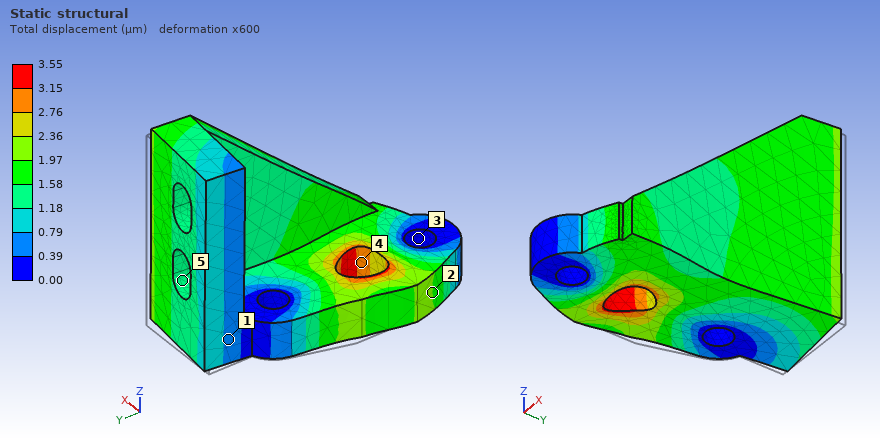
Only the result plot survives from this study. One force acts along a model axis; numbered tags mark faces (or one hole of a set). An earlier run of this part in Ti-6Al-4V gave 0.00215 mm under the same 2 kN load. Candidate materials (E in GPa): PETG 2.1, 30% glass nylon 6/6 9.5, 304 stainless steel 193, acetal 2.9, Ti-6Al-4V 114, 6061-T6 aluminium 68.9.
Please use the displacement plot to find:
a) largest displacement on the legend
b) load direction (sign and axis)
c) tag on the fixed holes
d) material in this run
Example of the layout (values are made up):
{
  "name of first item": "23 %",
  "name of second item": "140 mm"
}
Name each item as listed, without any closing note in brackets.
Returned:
{
  "largest displacement on the legend": "3.55 µm",
  "load direction": "-Y",
  "tag on the fixed holes": "3",
  "material in this run": "6061-T6 aluminium"
}
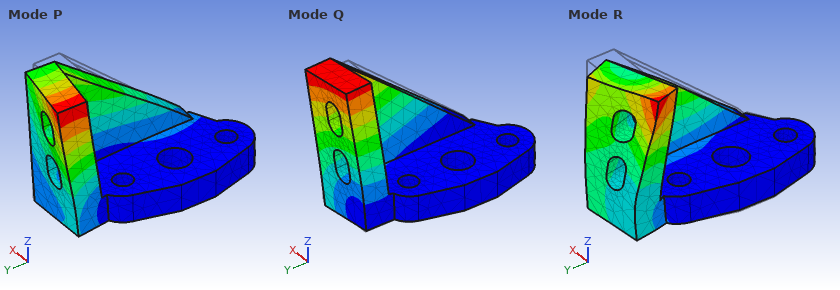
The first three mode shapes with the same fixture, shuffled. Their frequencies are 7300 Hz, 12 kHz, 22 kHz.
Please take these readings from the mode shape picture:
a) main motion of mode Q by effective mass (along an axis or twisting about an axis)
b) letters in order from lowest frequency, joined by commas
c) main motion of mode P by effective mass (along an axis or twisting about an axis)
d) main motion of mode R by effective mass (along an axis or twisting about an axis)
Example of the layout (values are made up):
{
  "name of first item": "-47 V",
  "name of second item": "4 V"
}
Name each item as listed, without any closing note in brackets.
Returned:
{
  "main motion of mode Q by effective mass": "along X",
  "letters in order from lowest frequency, joined by commas": "Q, P, R",
  "main motion of mode P by effective mass": "along Y",
  "main motion of mode R by effective mass": "along Z"
}
